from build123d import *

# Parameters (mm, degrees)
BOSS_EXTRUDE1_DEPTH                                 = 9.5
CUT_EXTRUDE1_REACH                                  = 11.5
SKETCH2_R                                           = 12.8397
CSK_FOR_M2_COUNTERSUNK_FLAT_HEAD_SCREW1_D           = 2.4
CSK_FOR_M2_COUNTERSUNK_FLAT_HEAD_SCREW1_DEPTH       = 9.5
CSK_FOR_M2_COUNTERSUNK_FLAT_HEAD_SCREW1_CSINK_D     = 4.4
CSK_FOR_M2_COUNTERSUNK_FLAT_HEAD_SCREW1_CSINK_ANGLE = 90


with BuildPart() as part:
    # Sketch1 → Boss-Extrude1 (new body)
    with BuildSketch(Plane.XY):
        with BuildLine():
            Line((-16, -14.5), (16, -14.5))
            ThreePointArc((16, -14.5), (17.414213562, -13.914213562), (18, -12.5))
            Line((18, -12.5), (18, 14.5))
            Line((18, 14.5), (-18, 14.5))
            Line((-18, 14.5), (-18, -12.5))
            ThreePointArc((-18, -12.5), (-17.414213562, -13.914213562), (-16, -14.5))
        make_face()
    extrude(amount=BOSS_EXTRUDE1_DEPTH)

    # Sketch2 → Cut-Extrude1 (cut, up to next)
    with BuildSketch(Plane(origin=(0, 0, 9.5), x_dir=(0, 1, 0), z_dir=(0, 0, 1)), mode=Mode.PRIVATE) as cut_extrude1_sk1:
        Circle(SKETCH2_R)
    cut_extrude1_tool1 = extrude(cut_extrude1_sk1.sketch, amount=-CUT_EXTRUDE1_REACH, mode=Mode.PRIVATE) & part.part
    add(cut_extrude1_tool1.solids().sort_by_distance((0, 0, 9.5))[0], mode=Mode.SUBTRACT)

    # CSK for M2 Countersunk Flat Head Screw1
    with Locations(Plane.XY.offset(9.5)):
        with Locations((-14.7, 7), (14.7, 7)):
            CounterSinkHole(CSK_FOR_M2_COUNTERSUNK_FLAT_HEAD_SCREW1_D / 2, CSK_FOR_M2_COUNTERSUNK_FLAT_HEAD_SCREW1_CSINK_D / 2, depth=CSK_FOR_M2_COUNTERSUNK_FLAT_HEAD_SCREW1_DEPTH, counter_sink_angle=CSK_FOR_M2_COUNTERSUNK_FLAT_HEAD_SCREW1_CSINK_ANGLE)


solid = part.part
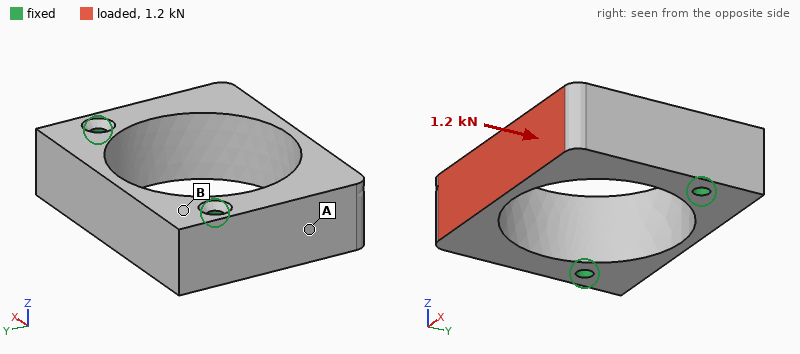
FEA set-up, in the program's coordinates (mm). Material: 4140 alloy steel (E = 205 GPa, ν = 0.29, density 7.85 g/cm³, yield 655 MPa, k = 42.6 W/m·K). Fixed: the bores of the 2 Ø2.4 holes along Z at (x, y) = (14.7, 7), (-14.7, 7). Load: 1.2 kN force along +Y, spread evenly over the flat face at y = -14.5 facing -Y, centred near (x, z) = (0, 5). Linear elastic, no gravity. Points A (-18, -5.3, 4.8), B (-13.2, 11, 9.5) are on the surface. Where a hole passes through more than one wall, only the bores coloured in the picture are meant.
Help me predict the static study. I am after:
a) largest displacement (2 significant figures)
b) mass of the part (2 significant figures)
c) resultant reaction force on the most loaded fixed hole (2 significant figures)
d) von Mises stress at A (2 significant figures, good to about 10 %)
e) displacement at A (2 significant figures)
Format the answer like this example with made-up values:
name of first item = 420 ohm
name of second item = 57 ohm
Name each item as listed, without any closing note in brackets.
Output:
largest displacement = 7.8 µm
mass of the part = 38 g
resultant reaction force on the most loaded fixed hole = 680 N
von Mises stress at A = 16 MPa
displacement at A = 1.8 µm
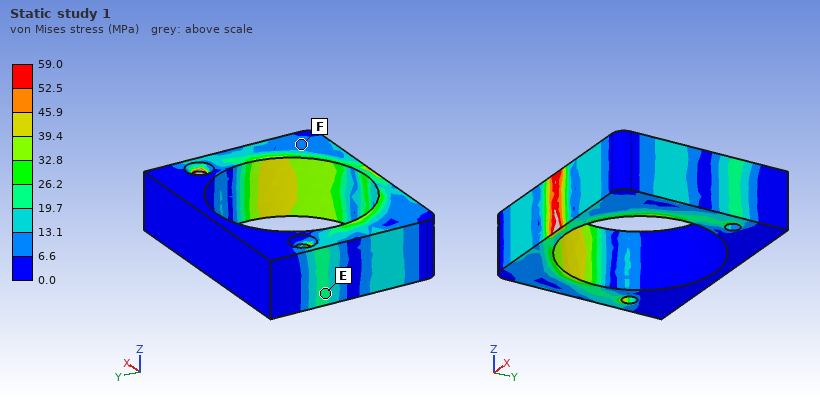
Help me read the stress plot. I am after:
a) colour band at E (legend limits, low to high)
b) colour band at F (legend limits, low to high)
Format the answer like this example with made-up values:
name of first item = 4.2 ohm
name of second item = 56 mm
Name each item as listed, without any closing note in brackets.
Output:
colour band at E = 19.7 to 26.2 MPa
colour band at F = 6.6 to 13.1 MPa
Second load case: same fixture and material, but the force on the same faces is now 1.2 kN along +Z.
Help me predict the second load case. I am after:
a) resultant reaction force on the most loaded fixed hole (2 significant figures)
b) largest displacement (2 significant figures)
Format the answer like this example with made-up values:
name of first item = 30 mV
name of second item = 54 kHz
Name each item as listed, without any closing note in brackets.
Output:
resultant reaction force on the most loaded fixed hole = 600 N
largest displacement = 40 µm
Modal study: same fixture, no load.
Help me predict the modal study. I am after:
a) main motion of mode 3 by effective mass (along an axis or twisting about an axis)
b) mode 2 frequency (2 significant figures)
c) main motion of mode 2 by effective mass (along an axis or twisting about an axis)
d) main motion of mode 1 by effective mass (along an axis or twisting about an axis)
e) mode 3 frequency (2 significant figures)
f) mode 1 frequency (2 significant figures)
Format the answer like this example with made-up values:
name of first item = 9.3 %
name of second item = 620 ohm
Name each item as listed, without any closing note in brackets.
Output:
main motion of mode 3 by effective mass = twisting about Y
mode 2 frequency = 9800 Hz
main motion of mode 2 by effective mass = along Z
main motion of mode 1 by effective mass = along X
mode 3 frequency = 15 kHz
mode 1 frequency = 8900 Hz
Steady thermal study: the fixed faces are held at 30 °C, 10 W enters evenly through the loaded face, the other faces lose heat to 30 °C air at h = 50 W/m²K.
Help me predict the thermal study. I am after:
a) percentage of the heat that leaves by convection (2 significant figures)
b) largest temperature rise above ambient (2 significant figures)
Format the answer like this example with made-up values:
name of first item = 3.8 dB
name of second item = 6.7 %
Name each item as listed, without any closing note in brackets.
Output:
percentage of the heat that leaves by convection = 18 %
largest temperature rise above ambient = 46 K
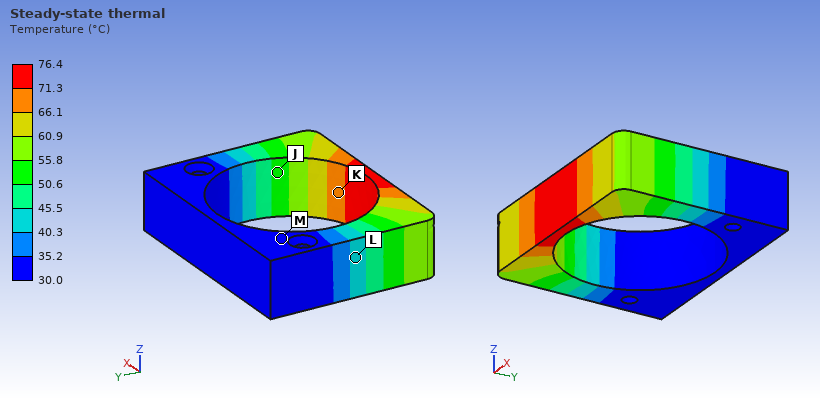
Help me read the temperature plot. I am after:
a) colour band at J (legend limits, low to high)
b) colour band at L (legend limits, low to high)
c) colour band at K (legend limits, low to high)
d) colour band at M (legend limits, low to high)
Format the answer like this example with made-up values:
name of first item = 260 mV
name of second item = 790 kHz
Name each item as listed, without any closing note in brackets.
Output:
colour band at J = 50.6 to 55.8 °C
colour band at L = 40.3 to 45.5 °C
colour band at K = 66.1 to 71.3 °C
colour band at M = 30.0 to 35.2 °C
